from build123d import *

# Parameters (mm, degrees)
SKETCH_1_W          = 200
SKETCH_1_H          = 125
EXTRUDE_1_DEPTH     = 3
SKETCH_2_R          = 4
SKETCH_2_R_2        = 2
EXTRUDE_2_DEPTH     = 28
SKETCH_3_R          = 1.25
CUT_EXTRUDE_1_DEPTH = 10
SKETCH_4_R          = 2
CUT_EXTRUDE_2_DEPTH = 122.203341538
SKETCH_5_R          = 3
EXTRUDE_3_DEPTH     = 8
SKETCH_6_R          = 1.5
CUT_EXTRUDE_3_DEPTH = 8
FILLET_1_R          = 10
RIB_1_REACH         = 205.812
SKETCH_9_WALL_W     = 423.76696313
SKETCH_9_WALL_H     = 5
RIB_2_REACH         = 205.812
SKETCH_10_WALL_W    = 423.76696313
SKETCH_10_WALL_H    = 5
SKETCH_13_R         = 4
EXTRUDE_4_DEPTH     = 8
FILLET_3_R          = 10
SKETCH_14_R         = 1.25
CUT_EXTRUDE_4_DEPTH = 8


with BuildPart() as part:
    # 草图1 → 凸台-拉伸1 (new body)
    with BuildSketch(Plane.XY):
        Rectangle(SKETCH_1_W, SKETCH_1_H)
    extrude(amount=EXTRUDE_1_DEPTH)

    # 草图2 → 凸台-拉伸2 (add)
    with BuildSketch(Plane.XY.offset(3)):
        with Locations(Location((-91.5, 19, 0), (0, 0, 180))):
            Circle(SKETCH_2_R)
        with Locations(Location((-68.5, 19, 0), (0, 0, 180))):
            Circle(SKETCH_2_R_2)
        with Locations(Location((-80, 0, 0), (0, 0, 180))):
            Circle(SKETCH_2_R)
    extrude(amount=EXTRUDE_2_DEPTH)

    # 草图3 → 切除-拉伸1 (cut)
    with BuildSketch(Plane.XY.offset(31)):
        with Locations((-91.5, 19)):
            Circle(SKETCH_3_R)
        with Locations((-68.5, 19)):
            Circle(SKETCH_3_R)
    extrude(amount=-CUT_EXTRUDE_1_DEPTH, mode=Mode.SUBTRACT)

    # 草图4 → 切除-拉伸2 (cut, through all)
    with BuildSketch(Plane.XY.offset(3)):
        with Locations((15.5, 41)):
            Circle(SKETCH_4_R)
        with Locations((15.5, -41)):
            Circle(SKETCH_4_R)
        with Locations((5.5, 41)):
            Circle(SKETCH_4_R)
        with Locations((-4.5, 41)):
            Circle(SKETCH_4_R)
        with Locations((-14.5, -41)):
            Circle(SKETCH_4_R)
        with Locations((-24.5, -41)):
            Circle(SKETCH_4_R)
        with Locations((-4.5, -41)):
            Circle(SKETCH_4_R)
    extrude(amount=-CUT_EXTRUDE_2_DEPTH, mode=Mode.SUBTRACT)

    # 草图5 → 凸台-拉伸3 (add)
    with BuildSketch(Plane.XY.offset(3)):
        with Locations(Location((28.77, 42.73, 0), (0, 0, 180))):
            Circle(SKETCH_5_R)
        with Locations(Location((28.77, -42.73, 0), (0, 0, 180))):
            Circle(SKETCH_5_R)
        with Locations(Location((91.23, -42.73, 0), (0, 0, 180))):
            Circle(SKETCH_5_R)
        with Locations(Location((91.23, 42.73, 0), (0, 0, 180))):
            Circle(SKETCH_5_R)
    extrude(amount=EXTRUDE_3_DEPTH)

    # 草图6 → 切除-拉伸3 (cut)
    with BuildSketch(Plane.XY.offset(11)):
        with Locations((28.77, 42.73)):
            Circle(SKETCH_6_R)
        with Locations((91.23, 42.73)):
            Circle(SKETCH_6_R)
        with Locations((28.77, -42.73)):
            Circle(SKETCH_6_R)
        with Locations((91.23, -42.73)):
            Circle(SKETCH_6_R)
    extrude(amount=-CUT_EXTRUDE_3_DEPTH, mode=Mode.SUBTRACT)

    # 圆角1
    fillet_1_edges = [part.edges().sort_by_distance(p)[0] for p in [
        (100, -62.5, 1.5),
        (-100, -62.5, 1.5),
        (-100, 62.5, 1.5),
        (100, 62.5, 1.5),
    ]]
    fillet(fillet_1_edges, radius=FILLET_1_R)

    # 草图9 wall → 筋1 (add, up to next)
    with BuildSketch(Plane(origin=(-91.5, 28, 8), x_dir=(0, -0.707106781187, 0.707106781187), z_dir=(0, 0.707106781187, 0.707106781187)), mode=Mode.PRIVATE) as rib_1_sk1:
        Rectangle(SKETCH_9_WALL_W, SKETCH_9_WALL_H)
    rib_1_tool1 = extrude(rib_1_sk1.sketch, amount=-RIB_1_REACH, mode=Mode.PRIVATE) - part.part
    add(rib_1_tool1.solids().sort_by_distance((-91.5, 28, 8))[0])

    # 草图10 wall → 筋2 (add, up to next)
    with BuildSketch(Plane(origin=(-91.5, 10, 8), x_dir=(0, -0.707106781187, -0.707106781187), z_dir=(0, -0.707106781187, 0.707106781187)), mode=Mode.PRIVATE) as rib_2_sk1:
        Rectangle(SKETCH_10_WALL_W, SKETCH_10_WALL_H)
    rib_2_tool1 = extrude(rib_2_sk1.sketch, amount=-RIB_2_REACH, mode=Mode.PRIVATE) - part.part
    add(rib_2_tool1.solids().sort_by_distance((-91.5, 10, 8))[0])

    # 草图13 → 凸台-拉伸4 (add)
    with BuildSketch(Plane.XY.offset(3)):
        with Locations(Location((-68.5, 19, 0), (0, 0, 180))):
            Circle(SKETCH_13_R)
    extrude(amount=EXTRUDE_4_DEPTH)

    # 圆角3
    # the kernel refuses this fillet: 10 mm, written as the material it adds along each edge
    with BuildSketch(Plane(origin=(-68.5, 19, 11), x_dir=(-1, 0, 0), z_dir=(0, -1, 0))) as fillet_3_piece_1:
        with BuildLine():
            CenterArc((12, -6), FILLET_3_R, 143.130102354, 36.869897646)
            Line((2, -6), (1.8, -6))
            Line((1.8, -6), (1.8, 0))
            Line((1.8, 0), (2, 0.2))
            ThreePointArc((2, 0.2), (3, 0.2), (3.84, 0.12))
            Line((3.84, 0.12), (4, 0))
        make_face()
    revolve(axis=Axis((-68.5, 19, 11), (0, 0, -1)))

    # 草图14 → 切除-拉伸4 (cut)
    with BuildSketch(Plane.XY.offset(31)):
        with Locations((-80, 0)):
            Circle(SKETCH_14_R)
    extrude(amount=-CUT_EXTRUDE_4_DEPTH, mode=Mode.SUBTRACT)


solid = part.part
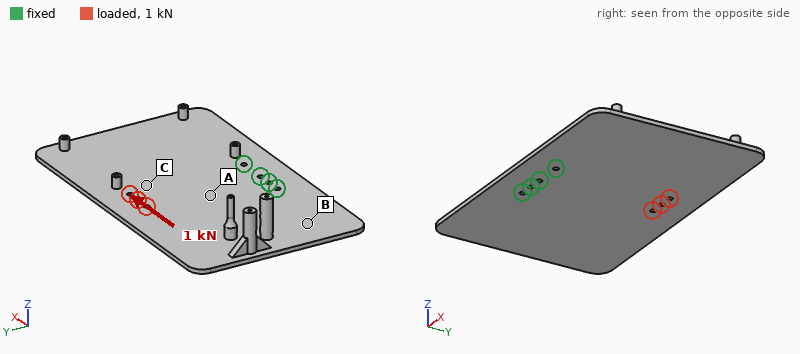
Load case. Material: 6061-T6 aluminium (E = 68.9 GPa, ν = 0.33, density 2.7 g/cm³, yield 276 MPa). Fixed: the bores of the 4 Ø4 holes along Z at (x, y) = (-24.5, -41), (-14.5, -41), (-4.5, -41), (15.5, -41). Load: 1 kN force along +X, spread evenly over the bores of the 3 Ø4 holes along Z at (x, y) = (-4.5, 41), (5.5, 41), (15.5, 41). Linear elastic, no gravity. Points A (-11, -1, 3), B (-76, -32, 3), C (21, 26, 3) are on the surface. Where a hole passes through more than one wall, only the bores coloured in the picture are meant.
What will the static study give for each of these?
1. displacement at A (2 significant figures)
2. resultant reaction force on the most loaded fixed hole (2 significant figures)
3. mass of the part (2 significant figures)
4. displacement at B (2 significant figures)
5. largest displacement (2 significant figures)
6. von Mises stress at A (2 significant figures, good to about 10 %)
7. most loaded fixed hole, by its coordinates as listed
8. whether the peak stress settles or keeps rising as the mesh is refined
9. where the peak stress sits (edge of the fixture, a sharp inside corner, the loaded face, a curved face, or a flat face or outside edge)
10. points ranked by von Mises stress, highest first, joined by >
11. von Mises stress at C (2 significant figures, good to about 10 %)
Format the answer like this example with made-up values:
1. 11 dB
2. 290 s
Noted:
1. 25 µm
2. 2.0 kN
3. 210 g
4. 37 µm
5. 84 µm
6. 11 MPa
7. (15.5, -41)
8. keeps rising
9. edge of the fixture
10. A > C > B
11. 6.5 MPa
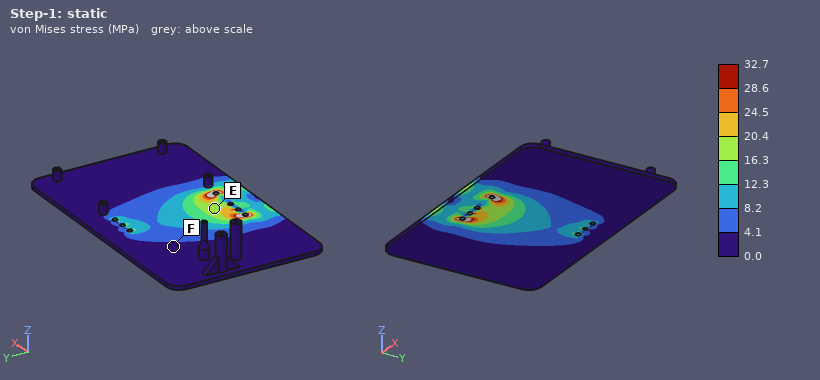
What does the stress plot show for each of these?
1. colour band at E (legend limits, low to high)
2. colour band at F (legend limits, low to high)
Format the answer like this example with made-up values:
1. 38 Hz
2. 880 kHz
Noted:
1. 16.3 to 20.4 MPa
2. 0.0 to 4.1 MPa
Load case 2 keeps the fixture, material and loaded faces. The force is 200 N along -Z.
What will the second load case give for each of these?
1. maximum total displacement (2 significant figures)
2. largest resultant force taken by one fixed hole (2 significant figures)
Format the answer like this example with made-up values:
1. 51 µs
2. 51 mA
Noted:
1. 2.7 mm
2. 80 N
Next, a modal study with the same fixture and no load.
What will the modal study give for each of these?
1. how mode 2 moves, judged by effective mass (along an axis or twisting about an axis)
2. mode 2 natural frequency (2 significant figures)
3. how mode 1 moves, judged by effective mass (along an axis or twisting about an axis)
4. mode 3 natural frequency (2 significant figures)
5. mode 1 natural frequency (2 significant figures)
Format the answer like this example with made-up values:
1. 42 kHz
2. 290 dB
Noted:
1. twisting about Y
2. 190 Hz
3. along Z
4. 350 Hz
5. 170 Hz
